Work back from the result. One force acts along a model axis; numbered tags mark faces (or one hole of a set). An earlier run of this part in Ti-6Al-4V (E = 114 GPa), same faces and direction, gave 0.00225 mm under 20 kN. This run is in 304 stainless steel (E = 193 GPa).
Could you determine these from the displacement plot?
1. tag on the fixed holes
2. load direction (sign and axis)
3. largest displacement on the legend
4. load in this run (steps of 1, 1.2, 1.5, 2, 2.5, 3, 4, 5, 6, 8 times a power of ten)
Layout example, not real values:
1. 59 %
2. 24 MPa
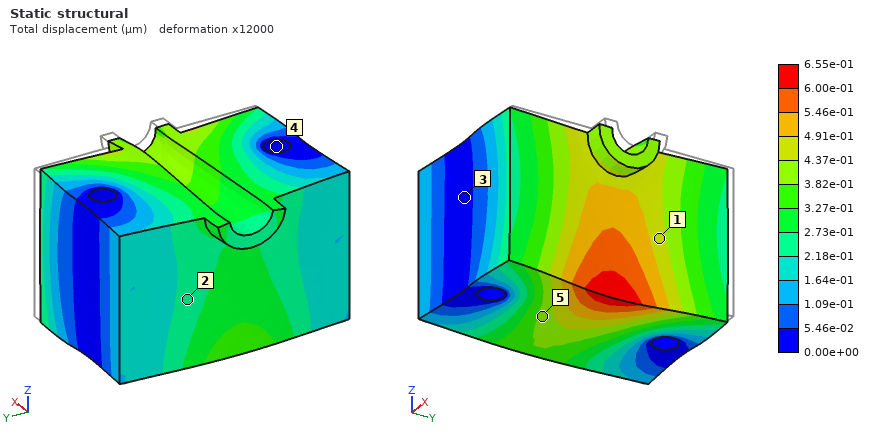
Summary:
1. 4
2. -X
3. 6.55e-01 µm
4. 10 kN
